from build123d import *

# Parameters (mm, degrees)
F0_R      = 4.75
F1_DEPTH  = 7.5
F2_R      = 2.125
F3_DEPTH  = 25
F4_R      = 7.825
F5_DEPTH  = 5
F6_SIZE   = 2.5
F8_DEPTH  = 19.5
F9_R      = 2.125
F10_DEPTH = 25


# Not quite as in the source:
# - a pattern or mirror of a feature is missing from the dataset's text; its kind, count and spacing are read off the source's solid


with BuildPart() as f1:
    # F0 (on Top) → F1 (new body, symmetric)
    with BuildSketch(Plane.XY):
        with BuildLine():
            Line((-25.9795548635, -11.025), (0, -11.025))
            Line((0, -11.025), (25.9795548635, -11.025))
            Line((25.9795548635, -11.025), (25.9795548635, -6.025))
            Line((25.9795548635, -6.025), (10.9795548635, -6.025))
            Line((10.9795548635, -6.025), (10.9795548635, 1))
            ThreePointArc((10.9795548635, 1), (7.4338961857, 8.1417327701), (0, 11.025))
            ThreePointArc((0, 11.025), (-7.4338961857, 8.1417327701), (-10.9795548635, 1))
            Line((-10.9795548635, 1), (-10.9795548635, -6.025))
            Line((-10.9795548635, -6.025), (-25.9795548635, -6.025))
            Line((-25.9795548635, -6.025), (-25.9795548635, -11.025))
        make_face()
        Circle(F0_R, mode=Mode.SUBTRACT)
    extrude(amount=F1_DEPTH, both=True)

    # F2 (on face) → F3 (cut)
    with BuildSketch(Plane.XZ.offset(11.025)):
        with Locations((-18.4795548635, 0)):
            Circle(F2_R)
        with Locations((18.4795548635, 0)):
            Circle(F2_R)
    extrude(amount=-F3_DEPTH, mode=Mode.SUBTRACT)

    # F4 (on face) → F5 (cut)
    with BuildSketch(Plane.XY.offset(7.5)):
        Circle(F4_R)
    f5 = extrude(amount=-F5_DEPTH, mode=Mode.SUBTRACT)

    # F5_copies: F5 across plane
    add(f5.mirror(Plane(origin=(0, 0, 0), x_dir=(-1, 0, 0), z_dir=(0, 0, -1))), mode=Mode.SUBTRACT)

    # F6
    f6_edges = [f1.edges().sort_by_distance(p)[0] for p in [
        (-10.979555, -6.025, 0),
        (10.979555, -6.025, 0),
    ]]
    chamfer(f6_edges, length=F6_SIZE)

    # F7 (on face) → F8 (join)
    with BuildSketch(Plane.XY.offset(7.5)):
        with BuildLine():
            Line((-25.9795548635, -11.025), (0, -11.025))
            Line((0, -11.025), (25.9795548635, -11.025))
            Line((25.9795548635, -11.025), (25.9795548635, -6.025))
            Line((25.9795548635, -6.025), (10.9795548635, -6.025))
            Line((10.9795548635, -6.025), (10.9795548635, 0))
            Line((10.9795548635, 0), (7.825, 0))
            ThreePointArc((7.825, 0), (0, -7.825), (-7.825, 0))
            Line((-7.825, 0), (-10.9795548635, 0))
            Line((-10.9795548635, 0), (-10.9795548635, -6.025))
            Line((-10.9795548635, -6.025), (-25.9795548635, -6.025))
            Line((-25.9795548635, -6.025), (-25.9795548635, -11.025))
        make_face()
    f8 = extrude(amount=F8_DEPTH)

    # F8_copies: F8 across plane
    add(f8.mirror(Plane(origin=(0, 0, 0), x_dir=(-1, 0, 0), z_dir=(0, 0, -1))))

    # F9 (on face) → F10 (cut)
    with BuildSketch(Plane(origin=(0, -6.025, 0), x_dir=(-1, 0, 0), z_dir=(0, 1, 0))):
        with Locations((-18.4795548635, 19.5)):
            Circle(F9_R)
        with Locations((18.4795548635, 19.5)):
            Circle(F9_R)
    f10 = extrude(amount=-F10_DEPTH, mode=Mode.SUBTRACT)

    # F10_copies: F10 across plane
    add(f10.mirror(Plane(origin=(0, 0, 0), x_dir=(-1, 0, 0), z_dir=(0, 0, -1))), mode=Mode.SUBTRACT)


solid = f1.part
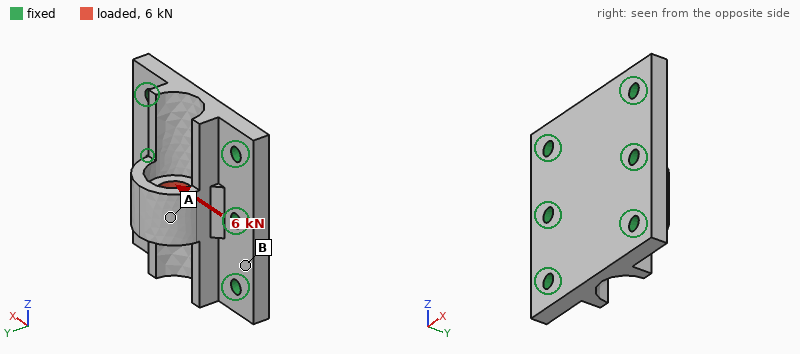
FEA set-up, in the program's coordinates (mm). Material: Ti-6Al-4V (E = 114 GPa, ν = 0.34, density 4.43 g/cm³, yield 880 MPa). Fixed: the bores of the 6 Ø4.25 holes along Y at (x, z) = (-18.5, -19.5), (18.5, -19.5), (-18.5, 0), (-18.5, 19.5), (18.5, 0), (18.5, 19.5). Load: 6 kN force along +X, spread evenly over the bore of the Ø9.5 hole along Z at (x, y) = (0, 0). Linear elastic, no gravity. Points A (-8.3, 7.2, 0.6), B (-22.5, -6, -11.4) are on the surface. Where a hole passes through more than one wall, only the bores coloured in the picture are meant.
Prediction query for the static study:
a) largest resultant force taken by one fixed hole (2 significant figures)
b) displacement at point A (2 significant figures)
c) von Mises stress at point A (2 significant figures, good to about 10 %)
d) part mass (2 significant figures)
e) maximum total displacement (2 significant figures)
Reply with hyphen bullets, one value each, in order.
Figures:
- 2.4 kN
- 22 µm
- 49 MPa
- 78 g
- 24 µm
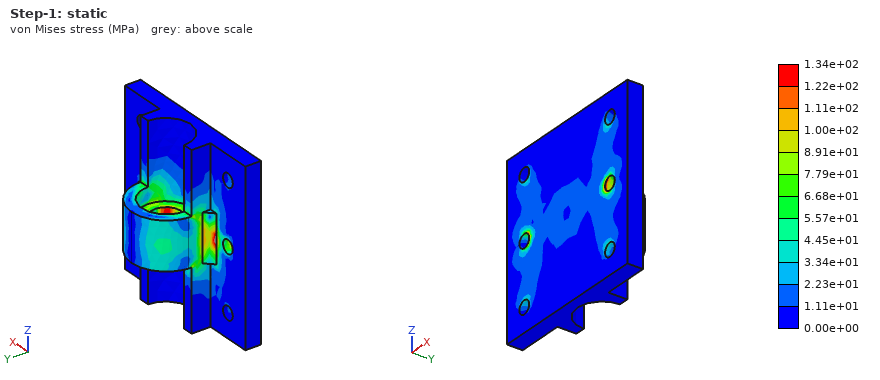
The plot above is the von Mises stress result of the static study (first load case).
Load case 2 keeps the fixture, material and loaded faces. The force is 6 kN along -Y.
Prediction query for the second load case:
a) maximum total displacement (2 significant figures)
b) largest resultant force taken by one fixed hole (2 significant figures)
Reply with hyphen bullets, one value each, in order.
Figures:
- 21 µm
- 2.0 kN
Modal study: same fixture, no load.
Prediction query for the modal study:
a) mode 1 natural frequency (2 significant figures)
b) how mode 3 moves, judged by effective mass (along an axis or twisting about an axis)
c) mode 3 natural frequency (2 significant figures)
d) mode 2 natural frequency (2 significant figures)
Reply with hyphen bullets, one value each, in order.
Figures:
- 16 kHz
- along X
- 22 kHz
- 16 kHz
